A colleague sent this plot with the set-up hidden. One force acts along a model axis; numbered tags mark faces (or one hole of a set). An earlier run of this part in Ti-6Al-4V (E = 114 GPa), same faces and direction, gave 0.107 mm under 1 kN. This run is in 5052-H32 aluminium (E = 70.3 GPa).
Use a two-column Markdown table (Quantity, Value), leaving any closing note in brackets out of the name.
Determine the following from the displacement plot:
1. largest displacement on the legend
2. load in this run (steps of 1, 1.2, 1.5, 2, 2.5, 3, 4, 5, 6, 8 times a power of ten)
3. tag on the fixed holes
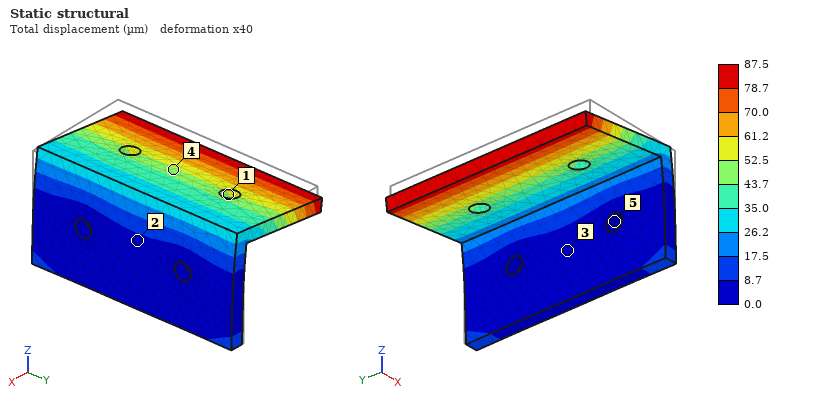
| Quantity | Value |
|---|---|
| largest displacement on the legend | 87.5 µm |
| load in this run | 500 N |
| tag on the fixed holes | 5 |
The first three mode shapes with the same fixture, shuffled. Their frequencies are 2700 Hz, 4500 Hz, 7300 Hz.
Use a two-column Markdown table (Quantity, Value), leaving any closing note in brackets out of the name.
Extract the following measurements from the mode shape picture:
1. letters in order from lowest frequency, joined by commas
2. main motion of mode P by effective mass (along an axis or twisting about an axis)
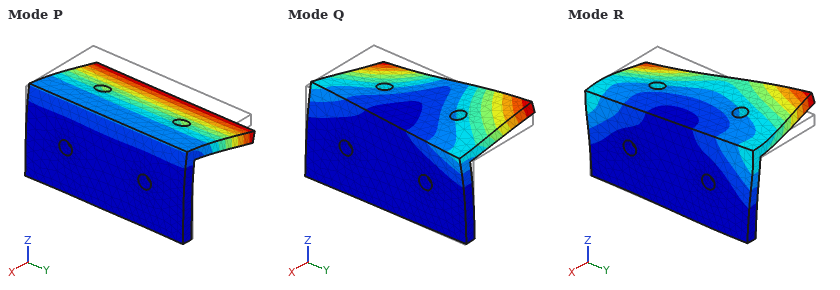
| Quantity | Value |
|---|---|
| letters in order from lowest frequency, joined by commas | P, Q, R |
| main motion of mode P by effective mass | along Z |
